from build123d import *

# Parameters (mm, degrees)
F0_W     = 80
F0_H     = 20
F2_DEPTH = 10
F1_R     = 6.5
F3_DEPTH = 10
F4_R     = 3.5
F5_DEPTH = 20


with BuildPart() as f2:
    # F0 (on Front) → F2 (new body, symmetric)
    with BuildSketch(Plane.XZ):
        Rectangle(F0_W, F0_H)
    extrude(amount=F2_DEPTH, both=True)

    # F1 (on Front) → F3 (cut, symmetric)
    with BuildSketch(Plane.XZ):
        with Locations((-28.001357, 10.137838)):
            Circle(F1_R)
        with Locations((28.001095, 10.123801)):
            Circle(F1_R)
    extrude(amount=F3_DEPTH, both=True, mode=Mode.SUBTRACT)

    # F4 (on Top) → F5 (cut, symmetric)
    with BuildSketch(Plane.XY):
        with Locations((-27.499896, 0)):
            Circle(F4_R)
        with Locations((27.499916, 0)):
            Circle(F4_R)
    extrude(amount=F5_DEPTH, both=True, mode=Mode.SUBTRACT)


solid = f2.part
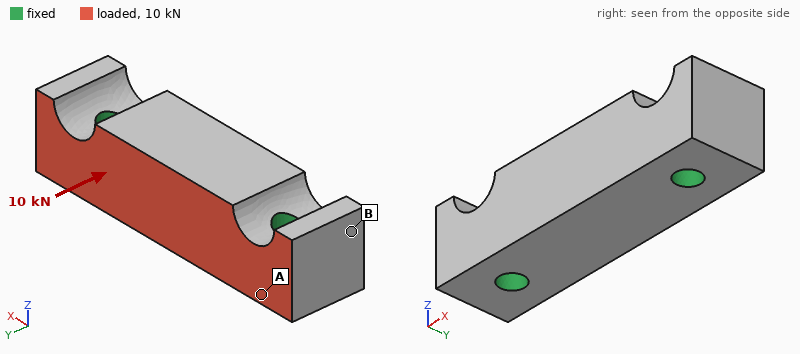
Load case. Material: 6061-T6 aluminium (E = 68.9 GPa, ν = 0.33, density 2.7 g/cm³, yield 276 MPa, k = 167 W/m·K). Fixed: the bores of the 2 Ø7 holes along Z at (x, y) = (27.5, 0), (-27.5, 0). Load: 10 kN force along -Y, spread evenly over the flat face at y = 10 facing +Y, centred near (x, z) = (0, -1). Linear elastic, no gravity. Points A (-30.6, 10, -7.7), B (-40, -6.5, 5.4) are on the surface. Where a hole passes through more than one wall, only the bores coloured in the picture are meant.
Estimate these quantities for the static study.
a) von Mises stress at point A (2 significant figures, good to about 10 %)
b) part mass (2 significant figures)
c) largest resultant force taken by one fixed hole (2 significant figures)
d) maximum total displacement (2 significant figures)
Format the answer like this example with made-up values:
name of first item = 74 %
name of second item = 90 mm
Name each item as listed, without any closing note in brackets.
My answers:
von Mises stress at point A = 14 MPa
part mass = 77 g
largest resultant force taken by one fixed hole = 5.0 kN
maximum total displacement = 14 µm
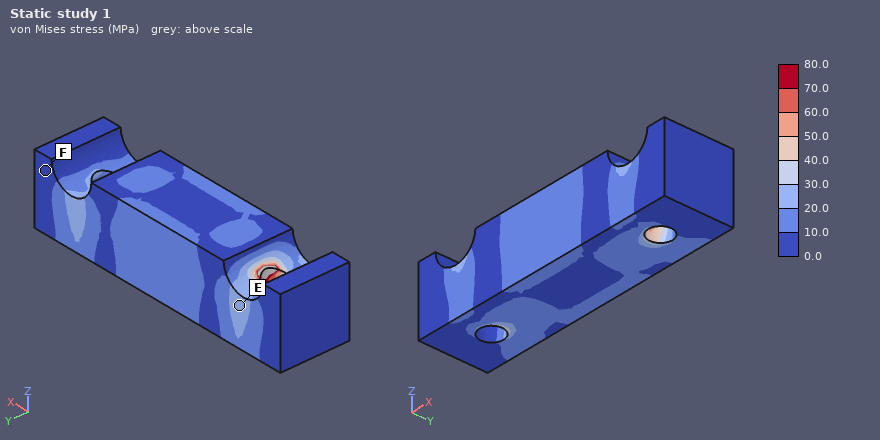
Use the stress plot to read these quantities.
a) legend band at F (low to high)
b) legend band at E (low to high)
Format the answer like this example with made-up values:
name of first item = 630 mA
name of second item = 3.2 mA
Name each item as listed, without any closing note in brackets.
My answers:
legend band at F = 0.0 to 10.0 MPa
legend band at E = 20.0 to 30.0 MPa
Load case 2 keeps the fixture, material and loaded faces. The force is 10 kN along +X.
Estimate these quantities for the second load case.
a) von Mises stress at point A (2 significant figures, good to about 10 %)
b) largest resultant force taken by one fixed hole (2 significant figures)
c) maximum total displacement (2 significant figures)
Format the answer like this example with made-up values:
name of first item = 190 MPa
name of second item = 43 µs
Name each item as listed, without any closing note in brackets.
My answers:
von Mises stress at point A = 14 MPa
largest resultant force taken by one fixed hole = 5.2 kN
maximum total displacement = 9.9 µm
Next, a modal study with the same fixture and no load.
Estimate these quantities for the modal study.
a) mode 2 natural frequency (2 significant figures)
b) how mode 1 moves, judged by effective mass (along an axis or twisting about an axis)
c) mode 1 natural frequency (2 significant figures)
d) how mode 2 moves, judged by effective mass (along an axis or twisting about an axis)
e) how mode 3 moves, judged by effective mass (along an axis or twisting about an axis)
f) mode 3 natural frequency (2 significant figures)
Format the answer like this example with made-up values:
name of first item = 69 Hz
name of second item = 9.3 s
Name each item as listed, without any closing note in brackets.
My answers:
mode 2 natural frequency = 19 kHz
how mode 1 moves, judged by effective mass = along Y
mode 1 natural frequency = 17 kHz
how mode 2 moves, judged by effective mass = along Z
how mode 3 moves, judged by effective mass = twisting about X
mode 3 natural frequency = 23 kHz
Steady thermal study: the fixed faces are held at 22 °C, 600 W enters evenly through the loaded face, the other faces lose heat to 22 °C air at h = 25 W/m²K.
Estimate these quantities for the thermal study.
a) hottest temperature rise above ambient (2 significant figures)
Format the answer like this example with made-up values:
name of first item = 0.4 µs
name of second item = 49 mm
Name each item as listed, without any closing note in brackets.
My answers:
hottest temperature rise above ambient = 68 K
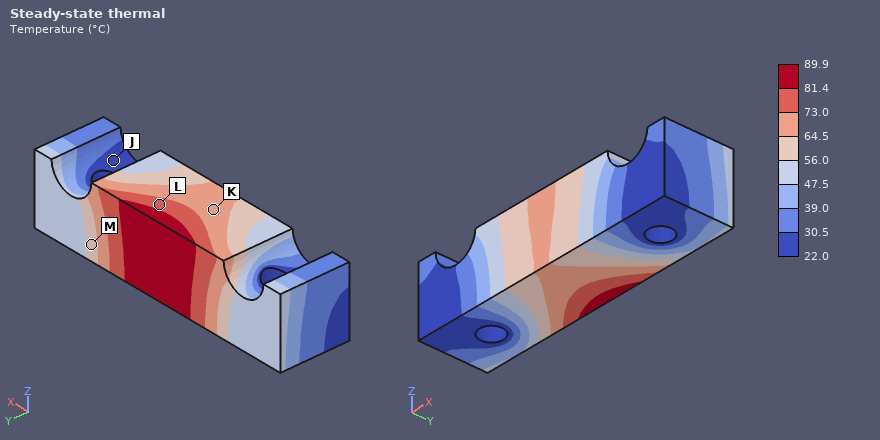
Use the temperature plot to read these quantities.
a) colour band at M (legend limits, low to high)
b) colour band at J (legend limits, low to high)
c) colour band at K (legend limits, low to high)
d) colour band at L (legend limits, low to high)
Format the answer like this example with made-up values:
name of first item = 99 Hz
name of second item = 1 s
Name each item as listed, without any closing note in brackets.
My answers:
colour band at M = 56.0 to 64.5 °C
colour band at J = 22.0 to 30.5 °C
colour band at K = 64.5 to 73.0 °C
colour band at L = 73.0 to 81.4 °C
